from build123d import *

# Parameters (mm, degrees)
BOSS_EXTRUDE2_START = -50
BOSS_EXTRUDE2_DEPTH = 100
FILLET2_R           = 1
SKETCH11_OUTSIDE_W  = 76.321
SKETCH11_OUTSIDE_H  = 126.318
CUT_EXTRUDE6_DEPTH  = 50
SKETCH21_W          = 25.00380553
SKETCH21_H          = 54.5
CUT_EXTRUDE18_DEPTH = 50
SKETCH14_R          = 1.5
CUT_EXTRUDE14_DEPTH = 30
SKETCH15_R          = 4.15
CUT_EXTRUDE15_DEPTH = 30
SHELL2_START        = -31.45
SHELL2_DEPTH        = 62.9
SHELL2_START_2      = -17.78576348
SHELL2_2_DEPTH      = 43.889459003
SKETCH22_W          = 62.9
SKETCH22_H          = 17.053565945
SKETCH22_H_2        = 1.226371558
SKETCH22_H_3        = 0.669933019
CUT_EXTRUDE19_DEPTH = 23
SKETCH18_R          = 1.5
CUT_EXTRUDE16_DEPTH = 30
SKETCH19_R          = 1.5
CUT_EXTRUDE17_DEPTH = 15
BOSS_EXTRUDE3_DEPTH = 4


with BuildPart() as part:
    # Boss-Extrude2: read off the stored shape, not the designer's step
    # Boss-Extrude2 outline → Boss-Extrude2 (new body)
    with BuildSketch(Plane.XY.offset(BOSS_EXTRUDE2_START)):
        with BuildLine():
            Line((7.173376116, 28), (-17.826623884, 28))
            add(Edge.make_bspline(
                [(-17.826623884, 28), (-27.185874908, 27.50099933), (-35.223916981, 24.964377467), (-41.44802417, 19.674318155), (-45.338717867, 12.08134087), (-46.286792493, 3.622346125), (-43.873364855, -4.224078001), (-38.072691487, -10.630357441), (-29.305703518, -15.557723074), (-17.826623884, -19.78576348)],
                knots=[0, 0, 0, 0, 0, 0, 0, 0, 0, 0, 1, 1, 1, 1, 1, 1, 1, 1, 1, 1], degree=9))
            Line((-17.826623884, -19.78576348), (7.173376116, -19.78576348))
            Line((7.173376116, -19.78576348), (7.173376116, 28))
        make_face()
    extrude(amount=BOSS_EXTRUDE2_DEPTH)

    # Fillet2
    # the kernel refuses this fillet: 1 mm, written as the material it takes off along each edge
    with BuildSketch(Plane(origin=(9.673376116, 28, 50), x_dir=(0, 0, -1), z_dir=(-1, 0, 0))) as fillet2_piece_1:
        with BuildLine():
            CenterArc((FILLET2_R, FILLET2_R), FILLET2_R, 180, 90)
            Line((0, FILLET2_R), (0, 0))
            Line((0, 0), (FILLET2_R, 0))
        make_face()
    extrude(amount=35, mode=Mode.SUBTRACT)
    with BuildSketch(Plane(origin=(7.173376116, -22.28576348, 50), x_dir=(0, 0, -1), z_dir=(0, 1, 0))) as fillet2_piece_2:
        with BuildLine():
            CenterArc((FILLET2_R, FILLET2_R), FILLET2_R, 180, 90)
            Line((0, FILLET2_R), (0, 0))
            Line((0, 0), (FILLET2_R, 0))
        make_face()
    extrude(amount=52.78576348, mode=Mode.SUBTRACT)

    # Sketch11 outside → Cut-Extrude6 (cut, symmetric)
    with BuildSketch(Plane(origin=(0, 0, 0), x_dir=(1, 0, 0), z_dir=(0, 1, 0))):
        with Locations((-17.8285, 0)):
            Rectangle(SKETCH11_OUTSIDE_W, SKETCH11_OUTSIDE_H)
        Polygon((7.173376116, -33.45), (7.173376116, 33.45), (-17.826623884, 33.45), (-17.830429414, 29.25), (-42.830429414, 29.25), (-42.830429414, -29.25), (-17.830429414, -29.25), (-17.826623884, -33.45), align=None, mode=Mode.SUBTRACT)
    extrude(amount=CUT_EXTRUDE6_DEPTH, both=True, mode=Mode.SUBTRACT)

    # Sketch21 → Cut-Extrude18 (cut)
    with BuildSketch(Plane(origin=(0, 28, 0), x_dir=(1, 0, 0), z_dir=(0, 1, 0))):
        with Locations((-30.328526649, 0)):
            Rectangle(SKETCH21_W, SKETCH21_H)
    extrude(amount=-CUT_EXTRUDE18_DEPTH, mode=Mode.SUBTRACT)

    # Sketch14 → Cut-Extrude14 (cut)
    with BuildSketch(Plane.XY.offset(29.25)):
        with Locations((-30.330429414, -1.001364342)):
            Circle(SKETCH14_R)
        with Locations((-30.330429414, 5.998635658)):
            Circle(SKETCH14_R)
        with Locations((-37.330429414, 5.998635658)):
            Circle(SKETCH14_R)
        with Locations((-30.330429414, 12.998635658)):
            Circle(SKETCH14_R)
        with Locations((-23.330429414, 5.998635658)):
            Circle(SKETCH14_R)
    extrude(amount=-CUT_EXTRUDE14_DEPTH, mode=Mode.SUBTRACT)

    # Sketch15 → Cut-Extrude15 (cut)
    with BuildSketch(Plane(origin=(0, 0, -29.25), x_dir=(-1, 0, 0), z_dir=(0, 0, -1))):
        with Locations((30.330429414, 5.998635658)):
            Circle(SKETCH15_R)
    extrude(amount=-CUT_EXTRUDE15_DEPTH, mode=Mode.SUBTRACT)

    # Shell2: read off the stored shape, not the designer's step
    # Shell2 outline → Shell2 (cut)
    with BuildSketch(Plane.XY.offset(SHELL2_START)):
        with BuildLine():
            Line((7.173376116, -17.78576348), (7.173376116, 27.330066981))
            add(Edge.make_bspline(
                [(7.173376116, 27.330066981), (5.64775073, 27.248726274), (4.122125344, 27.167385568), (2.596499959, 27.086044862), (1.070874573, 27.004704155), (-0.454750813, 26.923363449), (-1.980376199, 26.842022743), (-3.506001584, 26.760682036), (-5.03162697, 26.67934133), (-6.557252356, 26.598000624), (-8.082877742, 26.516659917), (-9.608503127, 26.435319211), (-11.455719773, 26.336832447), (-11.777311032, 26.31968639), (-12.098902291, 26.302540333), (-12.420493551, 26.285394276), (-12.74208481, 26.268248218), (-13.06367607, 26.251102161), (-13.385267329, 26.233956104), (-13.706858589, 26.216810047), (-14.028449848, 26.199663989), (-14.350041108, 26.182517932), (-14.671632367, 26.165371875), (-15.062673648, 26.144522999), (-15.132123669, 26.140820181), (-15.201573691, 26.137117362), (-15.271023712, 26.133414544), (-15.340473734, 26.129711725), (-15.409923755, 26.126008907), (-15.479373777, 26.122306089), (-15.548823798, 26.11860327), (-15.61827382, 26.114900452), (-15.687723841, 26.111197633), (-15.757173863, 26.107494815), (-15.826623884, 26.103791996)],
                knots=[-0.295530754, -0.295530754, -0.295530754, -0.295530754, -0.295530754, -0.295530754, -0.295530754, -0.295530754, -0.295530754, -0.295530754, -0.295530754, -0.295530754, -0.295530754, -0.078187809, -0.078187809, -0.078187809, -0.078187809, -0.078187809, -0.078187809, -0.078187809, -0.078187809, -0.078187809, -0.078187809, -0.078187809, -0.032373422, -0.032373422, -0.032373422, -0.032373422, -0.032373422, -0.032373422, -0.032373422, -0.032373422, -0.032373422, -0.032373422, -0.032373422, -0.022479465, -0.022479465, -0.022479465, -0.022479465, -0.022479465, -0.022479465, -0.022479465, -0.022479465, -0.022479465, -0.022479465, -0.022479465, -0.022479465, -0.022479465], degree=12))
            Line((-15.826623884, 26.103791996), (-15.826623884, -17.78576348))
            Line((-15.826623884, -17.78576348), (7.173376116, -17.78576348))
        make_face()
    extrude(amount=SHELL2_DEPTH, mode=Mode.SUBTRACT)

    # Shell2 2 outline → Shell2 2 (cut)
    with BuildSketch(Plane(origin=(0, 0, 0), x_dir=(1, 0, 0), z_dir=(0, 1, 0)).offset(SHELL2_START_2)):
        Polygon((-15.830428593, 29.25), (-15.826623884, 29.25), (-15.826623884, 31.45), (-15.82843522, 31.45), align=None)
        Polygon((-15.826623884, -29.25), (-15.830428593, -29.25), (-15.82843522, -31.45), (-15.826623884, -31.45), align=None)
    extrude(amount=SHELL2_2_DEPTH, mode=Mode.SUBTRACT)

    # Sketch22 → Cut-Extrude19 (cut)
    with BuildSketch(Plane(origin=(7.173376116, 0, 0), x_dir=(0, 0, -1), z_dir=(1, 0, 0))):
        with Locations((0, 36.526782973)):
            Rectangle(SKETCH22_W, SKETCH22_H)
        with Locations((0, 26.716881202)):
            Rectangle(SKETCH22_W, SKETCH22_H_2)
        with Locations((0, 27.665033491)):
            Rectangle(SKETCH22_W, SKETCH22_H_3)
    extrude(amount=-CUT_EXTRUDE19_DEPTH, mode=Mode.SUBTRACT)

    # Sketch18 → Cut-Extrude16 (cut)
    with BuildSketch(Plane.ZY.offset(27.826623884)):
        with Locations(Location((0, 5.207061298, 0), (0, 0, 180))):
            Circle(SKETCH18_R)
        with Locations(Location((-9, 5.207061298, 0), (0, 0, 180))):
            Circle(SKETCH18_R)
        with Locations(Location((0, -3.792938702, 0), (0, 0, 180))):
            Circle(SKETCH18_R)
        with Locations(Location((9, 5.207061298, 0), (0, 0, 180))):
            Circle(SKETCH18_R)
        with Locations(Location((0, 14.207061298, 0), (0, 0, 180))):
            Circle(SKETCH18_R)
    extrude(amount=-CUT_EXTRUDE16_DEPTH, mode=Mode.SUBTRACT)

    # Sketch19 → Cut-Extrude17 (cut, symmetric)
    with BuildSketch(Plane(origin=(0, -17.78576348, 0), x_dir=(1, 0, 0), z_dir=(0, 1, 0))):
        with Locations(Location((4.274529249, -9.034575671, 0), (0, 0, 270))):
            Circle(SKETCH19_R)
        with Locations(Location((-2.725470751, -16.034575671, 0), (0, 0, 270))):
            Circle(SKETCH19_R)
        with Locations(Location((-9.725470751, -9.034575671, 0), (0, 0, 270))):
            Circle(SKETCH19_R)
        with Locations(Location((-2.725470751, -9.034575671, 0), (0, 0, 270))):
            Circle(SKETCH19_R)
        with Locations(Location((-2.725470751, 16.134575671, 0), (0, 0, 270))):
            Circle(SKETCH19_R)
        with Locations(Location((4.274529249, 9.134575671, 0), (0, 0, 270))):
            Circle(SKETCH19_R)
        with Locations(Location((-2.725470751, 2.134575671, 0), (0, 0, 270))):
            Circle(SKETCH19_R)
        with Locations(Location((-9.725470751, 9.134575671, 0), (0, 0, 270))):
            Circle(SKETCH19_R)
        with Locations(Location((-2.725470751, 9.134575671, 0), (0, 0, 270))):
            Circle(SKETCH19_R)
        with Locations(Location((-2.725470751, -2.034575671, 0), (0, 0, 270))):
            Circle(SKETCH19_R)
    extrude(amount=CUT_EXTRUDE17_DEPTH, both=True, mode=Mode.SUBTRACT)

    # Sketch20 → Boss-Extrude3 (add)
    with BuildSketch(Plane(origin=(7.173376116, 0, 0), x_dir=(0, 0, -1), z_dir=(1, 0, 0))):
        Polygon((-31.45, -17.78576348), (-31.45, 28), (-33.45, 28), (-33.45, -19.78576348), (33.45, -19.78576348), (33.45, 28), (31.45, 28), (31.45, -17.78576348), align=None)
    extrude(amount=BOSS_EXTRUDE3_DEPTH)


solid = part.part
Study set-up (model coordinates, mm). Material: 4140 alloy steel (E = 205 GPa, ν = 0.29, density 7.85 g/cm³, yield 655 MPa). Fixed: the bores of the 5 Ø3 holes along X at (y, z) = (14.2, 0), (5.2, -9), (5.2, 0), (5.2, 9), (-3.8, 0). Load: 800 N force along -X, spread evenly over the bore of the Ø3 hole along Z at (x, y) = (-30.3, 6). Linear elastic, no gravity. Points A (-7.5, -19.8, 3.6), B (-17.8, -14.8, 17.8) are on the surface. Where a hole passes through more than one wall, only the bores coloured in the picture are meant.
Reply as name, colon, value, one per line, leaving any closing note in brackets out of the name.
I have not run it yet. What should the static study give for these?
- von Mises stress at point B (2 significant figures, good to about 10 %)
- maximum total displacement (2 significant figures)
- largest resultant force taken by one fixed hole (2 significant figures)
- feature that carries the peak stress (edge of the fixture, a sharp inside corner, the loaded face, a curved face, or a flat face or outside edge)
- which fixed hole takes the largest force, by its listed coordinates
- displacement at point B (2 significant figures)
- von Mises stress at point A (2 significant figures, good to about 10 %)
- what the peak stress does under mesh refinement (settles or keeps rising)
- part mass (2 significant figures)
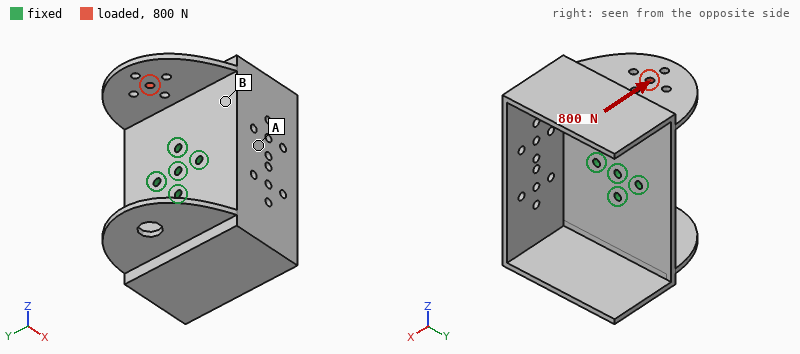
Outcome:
von Mises stress at point B: 100 MPa
maximum total displacement: 0.51 mm
largest resultant force taken by one fixed hole: 1.1 kN
feature that carries the peak stress: edge of the fixture
which fixed hole takes the largest force, by its listed coordinates: (5.2, 9)
displacement at point B: 0.13 mm
von Mises stress at point A: 37 MPa
what the peak stress does under mesh refinement: keeps rising
part mass: 140 g
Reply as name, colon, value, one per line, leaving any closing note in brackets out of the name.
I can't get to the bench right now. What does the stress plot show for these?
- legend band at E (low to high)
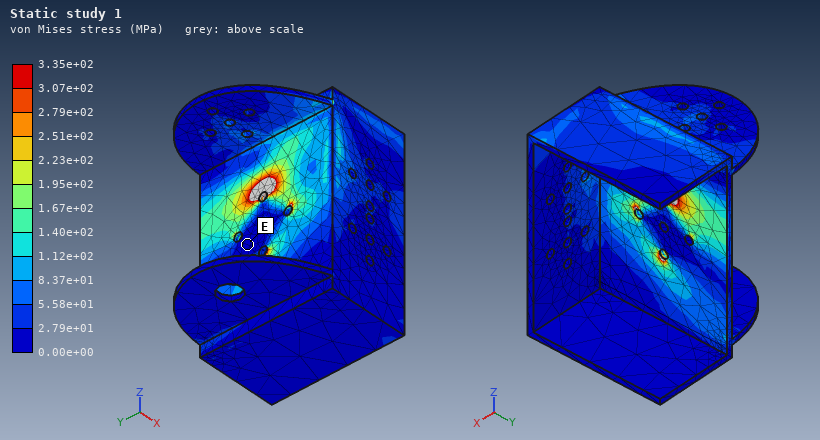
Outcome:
legend band at E: 0.00e+00 to 2.79e+01 MPa
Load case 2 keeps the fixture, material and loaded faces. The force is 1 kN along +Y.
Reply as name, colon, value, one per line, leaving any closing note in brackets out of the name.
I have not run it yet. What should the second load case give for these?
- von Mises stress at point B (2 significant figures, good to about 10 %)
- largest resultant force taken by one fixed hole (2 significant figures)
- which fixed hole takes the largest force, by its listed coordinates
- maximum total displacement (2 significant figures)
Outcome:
von Mises stress at point B: 49 MPa
largest resultant force taken by one fixed hole: 1.1 kN
which fixed hole takes the largest force, by its listed coordinates: (5.2, 9)
maximum total displacement: 0.47 mm
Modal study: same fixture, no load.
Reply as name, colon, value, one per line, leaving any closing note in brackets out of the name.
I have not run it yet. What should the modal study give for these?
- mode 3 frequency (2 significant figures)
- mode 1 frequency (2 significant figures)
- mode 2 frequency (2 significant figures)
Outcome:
mode 3 frequency: 1200 Hz
mode 1 frequency: 750 Hz
mode 2 frequency: 970 Hz
